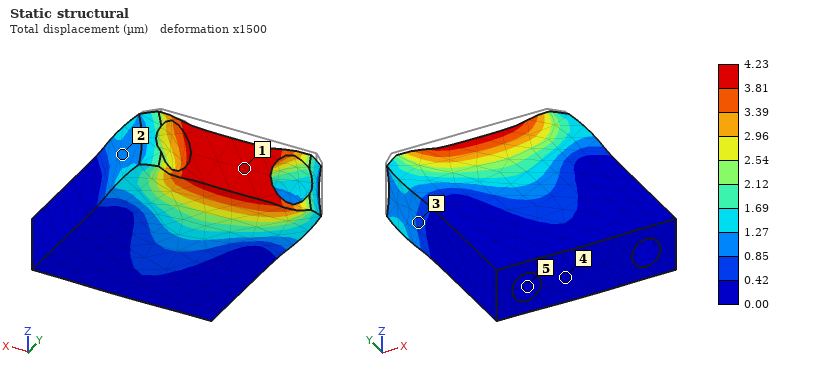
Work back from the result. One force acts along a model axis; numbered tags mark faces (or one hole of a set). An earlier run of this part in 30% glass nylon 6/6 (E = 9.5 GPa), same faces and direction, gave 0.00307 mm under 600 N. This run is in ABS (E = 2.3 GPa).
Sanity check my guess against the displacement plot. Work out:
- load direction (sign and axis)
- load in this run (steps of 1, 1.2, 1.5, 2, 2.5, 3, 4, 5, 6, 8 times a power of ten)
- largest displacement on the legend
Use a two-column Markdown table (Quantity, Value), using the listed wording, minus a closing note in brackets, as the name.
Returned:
| Quantity | Value |
|---|---|
| load direction | -Y |
| load in this run | 200 N |
| largest displacement on the legend | 4.23 µm |
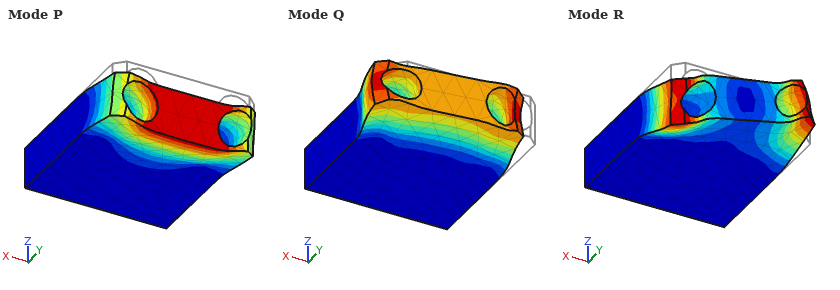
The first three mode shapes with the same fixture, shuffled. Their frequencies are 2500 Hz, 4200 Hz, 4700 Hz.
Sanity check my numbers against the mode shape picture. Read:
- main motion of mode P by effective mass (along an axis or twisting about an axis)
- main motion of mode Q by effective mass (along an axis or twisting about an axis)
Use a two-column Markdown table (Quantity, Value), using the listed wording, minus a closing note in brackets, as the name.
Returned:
| Quantity | Value |
|---|---|
| main motion of mode P by effective mass | along Z |
| main motion of mode Q by effective mass | along X |
